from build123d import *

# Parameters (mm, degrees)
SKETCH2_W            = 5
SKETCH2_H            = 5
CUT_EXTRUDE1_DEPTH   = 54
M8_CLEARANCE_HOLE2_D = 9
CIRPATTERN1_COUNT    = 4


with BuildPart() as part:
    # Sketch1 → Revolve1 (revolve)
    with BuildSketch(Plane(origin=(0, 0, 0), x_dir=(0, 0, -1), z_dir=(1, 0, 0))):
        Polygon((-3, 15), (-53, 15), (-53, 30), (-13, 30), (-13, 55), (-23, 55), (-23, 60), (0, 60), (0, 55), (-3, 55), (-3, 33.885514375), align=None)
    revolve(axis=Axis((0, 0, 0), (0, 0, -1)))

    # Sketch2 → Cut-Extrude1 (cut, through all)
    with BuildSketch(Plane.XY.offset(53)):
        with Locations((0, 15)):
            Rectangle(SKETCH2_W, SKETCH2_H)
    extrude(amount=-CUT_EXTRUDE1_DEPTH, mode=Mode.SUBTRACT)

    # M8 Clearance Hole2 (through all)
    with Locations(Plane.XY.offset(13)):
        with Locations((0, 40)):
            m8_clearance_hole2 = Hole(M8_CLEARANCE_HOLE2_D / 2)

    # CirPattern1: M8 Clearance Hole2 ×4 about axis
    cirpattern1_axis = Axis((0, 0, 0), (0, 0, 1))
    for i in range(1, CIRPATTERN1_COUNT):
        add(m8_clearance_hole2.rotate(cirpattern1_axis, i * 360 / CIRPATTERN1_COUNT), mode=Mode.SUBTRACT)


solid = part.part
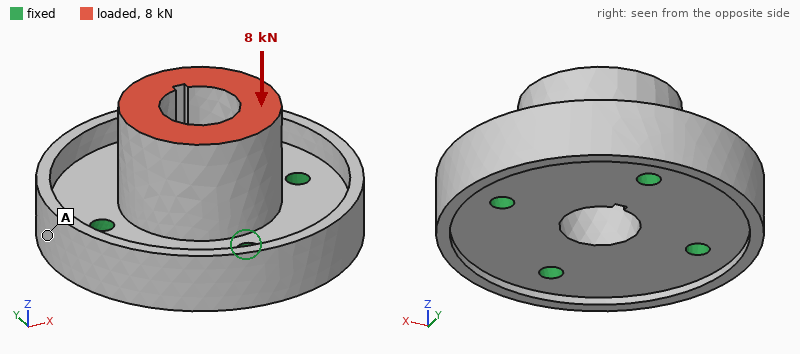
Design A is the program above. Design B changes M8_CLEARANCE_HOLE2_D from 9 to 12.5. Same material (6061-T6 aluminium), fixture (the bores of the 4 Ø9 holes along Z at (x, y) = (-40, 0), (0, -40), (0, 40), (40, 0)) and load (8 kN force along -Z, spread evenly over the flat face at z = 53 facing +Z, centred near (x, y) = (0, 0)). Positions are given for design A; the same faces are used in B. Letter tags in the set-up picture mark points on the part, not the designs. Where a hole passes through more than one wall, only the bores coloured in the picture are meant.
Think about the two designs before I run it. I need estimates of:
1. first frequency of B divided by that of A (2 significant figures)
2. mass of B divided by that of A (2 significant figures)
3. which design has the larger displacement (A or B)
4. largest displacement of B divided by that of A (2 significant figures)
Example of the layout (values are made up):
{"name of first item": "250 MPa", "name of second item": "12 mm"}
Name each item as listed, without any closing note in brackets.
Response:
{"first frequency of B divided by that of A": "1.1", "mass of B divided by that of A": "0.99", "which design has the larger displacement": "A", "largest displacement of B divided by that of A": "0.81"}
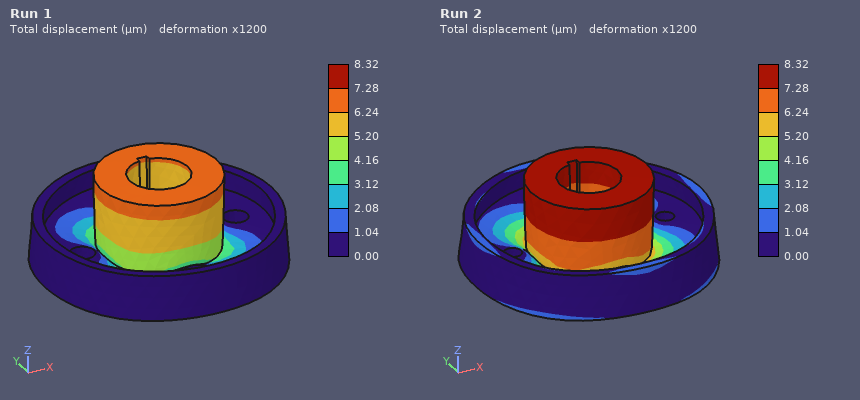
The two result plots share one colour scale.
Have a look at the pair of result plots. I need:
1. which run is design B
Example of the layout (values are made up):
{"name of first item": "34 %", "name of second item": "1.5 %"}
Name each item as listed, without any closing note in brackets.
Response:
{"which run is design B": "Run 1"}
